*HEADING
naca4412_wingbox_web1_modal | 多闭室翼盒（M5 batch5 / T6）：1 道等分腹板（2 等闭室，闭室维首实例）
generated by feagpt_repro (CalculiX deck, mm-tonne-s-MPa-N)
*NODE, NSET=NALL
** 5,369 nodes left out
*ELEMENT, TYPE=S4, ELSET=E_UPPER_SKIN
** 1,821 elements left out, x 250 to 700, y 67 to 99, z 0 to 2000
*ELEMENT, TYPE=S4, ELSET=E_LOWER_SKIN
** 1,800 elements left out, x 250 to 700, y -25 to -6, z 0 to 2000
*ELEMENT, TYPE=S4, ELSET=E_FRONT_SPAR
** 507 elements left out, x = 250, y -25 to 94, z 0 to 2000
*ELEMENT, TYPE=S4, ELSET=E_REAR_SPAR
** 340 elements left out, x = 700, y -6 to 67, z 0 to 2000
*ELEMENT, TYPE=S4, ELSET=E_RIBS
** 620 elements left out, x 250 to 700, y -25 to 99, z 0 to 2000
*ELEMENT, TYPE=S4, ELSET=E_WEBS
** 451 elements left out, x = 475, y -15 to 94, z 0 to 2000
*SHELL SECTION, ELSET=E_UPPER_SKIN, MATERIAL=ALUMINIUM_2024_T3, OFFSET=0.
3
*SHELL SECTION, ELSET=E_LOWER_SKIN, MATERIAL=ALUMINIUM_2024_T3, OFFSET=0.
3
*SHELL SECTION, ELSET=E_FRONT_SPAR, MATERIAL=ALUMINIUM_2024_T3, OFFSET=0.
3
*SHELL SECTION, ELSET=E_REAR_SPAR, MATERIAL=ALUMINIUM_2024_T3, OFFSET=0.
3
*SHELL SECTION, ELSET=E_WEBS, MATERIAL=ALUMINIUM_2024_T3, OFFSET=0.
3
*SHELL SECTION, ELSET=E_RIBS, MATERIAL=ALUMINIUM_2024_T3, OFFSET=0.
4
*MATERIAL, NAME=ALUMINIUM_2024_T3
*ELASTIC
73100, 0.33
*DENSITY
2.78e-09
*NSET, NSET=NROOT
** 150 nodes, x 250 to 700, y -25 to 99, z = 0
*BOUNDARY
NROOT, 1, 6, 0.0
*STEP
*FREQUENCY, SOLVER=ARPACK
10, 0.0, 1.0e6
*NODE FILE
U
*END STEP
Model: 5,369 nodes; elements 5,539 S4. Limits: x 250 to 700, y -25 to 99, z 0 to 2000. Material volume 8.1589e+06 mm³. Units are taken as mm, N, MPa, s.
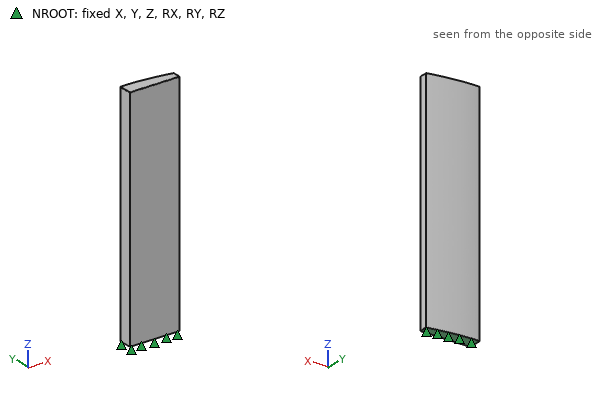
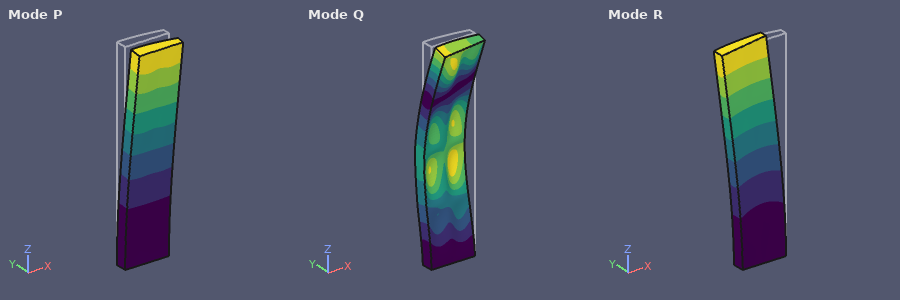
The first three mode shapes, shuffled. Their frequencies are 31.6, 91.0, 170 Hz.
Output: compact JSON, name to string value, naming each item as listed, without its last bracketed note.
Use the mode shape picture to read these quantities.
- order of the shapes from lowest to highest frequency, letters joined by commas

{"order of the shapes from lowest to highest frequency, letters joined by commas": "P, R, Q"}
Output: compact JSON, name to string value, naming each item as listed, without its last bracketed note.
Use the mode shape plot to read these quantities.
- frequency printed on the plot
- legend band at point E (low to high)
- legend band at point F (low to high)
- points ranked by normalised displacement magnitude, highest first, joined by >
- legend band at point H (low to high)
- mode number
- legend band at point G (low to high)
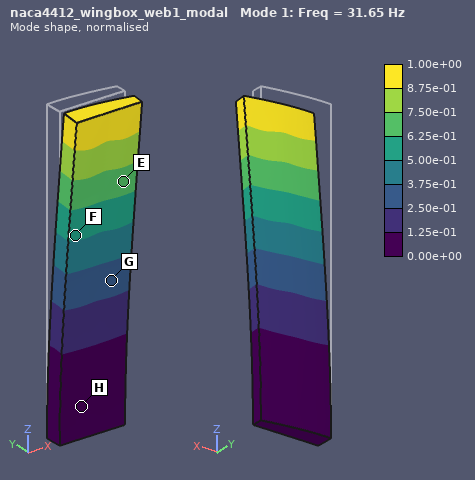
{"frequency printed on the plot": "31.65 Hz", "legend band at point E": "6.25e-01 to 7.50e-01", "legend band at point F": "5.00e-01 to 6.25e-01", "points ranked by normalised displacement magnitude, highest first, joined by >": "E > F > G > H", "legend band at point H": "0.00e+00 to 1.25e-01", "mode number": "1", "legend band at point G": "2.50e-01 to 3.75e-01"}
